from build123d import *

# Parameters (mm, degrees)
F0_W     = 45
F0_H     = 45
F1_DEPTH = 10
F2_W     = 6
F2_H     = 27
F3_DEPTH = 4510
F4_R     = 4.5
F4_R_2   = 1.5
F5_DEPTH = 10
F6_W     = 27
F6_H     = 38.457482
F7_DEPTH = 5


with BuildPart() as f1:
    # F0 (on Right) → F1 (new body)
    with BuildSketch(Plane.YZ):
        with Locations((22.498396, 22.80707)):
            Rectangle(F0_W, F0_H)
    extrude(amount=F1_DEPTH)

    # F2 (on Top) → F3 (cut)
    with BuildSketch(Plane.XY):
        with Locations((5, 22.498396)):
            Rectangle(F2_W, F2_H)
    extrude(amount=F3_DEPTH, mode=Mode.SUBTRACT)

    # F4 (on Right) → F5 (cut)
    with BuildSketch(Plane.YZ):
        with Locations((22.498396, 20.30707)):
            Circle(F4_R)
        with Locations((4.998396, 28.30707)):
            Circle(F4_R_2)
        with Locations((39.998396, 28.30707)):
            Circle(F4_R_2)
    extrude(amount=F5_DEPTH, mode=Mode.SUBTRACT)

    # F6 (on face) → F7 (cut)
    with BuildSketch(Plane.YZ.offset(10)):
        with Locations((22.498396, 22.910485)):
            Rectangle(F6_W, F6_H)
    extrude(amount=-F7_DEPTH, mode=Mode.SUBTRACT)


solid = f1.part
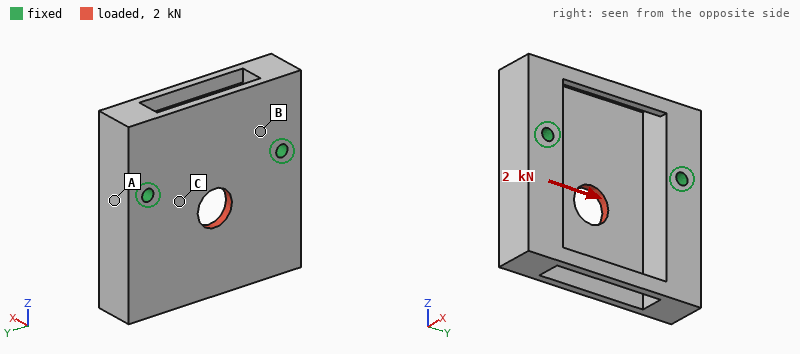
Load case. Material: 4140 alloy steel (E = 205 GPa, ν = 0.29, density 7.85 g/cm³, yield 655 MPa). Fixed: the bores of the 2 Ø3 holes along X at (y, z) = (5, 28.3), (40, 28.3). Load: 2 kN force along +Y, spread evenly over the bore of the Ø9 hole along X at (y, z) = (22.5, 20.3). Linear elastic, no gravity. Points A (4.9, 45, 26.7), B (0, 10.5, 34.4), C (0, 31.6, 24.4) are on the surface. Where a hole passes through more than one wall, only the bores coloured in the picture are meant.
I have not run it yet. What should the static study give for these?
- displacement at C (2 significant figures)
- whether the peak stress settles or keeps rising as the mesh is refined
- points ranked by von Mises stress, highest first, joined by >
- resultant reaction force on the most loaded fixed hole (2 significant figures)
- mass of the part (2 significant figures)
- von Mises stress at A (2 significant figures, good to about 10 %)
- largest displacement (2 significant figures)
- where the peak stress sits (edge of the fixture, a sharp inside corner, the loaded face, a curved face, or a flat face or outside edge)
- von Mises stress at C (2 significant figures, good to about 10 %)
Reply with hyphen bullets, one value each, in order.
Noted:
- 1.8 µm
- keeps rising
- C > A > B
- 1.1 kN
- 83 g
- 18 MPa
- 4.7 µm
- edge of the fixture
- 33 MPa
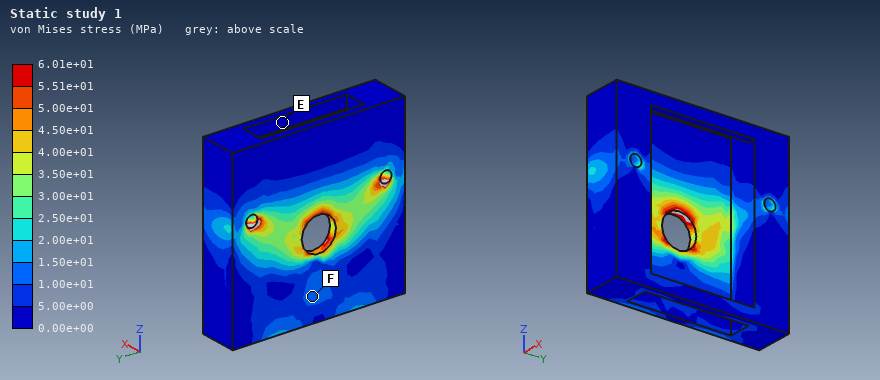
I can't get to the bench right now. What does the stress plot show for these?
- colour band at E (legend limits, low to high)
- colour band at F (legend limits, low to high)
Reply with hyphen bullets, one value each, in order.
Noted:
- 0.00e+00 to 5.00e+00 MPa
- 1.00e+01 to 1.50e+01 MPa
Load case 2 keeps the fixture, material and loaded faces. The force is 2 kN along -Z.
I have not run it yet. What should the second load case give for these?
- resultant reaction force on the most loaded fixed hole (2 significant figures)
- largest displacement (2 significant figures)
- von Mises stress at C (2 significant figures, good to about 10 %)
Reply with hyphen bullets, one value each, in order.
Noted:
- 1.0 kN
- 4.6 µm
- 27 MPa
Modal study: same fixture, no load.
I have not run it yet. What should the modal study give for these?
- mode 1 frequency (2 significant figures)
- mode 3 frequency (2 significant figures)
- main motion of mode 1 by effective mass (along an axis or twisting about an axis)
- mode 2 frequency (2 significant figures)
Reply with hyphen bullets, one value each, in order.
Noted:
- 7900 Hz
- 12 kHz
- along X
- 9300 Hz
